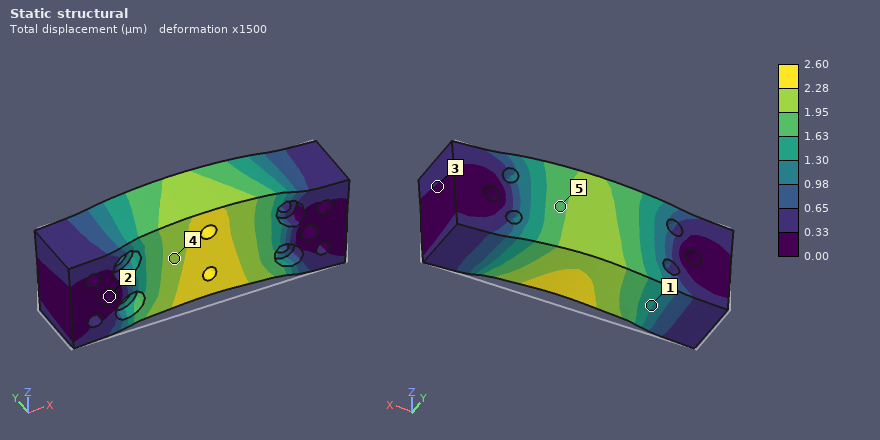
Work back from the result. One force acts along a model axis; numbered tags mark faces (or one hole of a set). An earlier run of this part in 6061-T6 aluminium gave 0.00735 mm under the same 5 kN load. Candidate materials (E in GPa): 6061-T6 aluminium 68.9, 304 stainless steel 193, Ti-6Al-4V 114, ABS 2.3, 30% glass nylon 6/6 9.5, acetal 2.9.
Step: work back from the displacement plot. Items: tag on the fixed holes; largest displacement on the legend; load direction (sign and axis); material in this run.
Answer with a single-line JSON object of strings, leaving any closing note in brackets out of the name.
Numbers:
{"tag on the fixed holes": "2", "largest displacement on the legend": "2.60 µm", "load direction": "+Z", "material in this run": "304 stainless steel"}
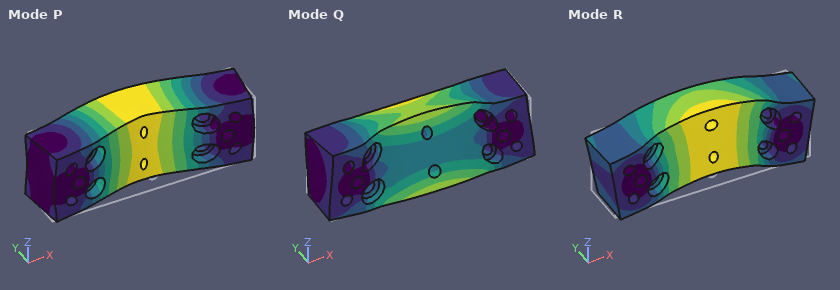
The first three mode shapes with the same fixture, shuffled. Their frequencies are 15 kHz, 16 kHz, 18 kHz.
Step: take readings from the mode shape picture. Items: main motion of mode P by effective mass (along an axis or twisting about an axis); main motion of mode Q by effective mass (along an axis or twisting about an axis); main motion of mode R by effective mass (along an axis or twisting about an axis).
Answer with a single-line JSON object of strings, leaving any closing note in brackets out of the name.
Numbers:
{"main motion of mode P by effective mass": "along Y", "main motion of mode Q by effective mass": "twisting about X", "main motion of mode R by effective mass": "along Z"}
